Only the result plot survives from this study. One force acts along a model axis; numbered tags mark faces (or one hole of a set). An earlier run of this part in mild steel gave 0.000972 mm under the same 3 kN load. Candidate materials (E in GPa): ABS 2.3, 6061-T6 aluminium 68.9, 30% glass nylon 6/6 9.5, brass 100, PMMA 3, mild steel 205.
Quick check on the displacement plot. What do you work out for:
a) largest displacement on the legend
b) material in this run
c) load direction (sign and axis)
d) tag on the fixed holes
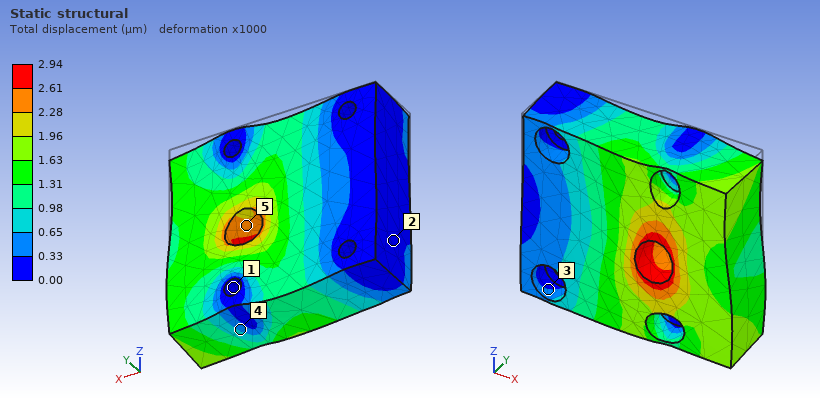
2.94 µm
6061-T6 aluminium
-Z
1
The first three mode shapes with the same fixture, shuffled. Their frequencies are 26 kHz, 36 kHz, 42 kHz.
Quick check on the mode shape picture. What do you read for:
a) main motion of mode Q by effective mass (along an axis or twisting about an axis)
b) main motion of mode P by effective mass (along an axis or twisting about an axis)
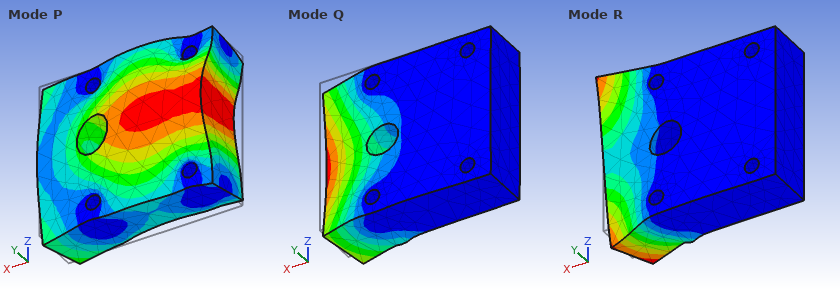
along Y
along Y
